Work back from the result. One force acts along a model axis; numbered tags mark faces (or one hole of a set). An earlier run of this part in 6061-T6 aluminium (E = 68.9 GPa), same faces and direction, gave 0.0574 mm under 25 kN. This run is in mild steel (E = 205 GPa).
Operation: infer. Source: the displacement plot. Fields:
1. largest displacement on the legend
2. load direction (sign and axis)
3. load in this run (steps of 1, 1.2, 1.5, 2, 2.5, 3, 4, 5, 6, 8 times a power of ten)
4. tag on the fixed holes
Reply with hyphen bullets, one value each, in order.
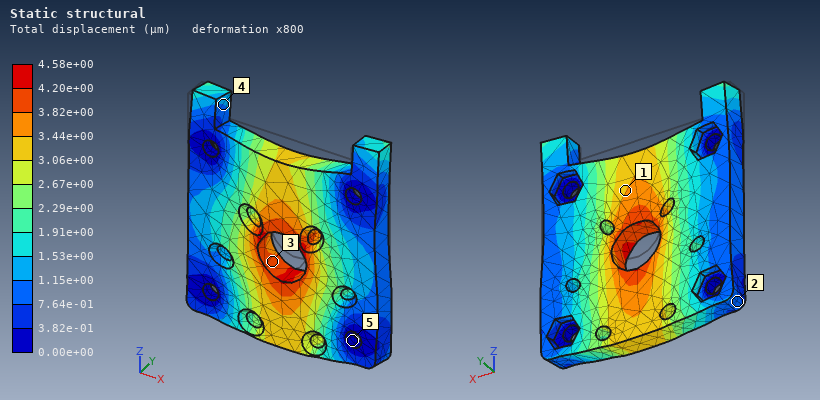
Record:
- 4.58e+00 µm
- -Z
- 6 kN
- 5
